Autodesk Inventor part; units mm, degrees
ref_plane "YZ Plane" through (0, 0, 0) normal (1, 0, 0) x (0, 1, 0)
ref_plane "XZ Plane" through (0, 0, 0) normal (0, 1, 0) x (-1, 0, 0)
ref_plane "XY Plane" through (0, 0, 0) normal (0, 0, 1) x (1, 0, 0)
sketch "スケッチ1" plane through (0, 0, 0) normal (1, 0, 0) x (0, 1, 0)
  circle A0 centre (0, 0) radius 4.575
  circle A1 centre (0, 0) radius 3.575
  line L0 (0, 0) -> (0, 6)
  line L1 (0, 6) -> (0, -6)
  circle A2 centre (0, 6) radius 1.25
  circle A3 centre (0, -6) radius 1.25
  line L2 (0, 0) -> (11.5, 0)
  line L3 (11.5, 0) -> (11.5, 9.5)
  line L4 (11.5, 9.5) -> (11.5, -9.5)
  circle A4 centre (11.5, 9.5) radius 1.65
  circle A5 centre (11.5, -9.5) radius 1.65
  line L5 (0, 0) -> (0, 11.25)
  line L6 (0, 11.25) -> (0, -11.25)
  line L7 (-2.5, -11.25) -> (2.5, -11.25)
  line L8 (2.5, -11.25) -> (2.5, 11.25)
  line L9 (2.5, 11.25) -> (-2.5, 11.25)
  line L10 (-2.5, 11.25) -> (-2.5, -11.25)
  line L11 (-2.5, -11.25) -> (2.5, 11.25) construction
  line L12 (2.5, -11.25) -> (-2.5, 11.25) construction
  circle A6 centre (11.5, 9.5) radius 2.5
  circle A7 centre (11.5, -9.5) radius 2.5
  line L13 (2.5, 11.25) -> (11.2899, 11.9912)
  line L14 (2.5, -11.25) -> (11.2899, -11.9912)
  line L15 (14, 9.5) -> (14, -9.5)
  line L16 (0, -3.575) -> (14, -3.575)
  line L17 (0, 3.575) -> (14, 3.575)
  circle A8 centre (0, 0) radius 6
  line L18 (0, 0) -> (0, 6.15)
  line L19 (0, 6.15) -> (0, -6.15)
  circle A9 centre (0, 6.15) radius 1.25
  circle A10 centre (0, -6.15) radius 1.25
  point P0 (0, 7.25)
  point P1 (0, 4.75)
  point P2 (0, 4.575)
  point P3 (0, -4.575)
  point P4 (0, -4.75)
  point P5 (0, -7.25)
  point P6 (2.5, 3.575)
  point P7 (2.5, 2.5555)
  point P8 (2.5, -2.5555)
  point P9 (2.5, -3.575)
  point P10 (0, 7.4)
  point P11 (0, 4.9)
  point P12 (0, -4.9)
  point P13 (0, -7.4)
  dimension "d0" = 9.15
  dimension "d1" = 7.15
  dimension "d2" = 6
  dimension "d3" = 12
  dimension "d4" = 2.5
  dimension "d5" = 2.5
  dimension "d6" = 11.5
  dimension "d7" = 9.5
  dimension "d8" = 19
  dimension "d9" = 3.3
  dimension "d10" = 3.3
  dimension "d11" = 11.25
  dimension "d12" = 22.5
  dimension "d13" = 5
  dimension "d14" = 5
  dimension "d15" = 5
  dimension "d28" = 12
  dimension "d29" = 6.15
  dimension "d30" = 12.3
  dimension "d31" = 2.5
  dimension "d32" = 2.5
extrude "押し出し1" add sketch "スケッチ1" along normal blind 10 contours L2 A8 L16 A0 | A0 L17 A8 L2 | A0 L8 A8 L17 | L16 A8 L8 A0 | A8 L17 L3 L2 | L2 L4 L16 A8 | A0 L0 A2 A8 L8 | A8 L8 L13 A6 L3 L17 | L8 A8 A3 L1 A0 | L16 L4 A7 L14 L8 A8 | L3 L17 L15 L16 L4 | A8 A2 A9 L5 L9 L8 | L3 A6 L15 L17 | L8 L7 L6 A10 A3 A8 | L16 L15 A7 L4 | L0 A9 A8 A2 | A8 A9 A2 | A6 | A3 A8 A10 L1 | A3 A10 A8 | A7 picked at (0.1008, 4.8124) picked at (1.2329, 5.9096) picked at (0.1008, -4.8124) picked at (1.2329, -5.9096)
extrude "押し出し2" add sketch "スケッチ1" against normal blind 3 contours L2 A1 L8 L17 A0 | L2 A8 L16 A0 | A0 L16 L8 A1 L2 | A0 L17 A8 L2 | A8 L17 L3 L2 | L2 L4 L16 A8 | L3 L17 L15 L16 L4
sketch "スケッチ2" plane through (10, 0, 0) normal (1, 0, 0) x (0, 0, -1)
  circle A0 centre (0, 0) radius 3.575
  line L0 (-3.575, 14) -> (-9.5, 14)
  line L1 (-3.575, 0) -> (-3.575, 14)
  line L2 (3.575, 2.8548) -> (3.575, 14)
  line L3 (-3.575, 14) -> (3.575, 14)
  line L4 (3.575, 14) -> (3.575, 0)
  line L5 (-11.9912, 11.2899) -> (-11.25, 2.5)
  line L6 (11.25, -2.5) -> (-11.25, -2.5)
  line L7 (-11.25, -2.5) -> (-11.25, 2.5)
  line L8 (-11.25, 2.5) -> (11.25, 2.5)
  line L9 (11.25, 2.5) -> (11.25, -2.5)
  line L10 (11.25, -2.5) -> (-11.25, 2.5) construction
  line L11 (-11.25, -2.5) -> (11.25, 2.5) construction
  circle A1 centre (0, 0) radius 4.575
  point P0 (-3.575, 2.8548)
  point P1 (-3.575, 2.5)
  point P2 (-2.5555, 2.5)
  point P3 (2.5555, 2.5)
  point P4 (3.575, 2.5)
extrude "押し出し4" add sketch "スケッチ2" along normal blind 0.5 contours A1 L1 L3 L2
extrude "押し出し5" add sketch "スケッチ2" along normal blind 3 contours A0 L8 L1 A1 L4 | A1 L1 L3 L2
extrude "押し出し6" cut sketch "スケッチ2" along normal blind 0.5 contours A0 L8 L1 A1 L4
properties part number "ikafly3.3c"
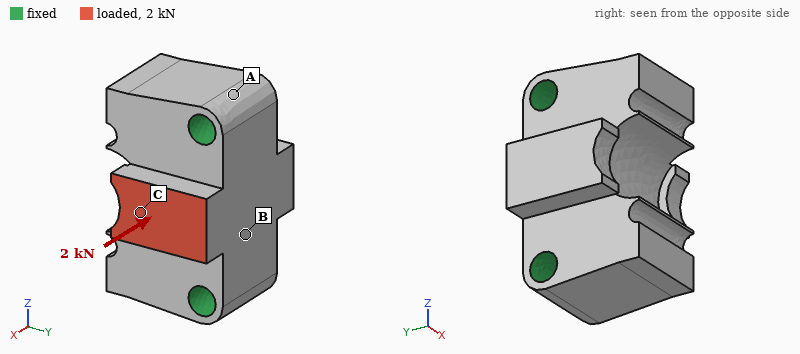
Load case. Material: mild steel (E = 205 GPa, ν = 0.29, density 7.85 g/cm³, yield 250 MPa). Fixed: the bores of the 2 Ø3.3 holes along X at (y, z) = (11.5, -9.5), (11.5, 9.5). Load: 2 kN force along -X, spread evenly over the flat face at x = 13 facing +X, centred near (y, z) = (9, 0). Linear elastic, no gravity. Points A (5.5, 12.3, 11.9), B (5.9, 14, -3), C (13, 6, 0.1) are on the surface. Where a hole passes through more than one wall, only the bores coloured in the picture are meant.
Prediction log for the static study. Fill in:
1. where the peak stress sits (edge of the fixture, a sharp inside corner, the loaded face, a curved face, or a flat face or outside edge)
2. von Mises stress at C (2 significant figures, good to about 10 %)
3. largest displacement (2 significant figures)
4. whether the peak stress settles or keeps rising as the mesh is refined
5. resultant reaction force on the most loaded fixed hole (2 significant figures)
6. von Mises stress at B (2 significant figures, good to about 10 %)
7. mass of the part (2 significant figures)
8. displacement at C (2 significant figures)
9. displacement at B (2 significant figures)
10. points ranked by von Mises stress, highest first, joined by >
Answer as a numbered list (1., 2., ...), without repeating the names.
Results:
1. a sharp inside corner
2. 30 MPa
3. 3.0 µm
4. keeps rising
5. 1.0 kN
6. 17 MPa
7. 25 g
8. 2.4 µm
9. 0.82 µm
10. C > B > A
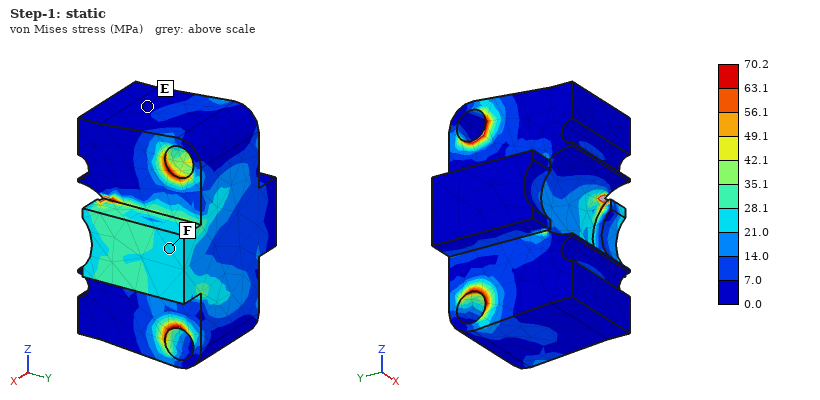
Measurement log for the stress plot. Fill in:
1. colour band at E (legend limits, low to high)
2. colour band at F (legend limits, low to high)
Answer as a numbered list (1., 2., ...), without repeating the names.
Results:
1. 0.0 to 7.0 MPa
2. 21.0 to 28.1 MPa
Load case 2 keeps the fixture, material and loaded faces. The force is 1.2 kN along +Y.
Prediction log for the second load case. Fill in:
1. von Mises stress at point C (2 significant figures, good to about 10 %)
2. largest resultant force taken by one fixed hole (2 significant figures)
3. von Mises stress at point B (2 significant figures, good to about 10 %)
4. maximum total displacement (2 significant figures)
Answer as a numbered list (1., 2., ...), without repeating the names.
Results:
1. 37 MPa
2. 690 N
3. 36 MPa
4. 6.2 µm
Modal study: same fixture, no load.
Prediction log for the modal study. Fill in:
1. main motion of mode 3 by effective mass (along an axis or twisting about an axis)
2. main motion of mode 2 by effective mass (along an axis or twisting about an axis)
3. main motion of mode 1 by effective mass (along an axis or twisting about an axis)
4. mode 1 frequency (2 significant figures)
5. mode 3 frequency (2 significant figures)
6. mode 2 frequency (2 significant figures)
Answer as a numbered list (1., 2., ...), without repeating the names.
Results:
1. twisting about Y
2. along Y
3. along X
4. 38 kHz
5. 59 kHz
6. 47 kHz
